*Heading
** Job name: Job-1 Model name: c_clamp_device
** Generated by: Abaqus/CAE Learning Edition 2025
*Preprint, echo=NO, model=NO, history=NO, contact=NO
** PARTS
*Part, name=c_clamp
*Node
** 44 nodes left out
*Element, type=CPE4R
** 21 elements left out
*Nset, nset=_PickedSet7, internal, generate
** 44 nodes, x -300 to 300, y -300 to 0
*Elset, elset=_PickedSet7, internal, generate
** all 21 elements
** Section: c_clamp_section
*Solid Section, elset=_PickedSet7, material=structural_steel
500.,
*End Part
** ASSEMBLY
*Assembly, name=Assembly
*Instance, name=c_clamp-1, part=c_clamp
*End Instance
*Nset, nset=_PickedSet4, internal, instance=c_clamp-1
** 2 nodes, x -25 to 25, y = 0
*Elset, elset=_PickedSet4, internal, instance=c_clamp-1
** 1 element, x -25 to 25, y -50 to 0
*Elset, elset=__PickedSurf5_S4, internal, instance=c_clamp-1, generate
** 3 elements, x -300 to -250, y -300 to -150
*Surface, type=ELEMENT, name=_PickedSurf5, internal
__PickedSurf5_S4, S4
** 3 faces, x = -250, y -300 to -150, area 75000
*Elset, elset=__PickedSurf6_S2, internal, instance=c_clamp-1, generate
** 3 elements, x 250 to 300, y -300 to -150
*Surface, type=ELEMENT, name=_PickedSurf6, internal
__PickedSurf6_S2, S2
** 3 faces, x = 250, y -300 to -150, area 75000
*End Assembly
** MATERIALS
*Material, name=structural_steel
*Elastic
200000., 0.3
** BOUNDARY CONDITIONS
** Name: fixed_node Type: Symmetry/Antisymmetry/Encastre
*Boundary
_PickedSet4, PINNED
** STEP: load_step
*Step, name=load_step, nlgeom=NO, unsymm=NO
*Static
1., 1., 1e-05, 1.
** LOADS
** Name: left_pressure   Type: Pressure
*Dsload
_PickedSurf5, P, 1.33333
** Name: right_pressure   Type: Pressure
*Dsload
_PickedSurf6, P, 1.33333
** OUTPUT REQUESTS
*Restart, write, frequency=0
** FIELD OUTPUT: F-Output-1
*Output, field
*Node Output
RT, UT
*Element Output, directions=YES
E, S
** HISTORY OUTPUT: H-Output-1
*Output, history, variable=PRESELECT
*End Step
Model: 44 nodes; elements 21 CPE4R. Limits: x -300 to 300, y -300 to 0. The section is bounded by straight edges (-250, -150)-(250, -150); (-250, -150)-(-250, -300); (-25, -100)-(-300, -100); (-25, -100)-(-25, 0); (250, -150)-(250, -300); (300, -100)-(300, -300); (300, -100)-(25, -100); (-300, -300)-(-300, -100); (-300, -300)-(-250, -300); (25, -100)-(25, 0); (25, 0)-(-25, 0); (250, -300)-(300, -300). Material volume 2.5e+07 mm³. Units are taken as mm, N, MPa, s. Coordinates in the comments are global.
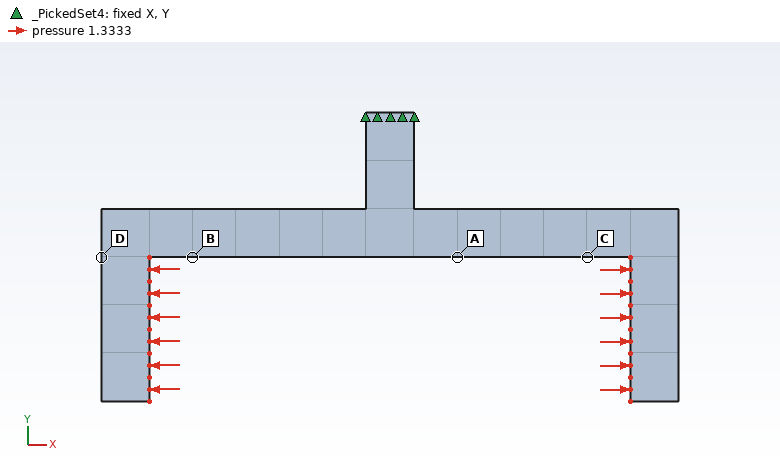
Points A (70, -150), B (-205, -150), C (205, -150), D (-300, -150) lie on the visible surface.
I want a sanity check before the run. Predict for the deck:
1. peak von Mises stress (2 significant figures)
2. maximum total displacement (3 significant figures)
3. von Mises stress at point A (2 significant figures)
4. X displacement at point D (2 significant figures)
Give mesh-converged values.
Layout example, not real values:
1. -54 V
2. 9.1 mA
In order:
1. 51 MPa
2. 0.595 mm
3. 46 MPa
4. -0.062 mm
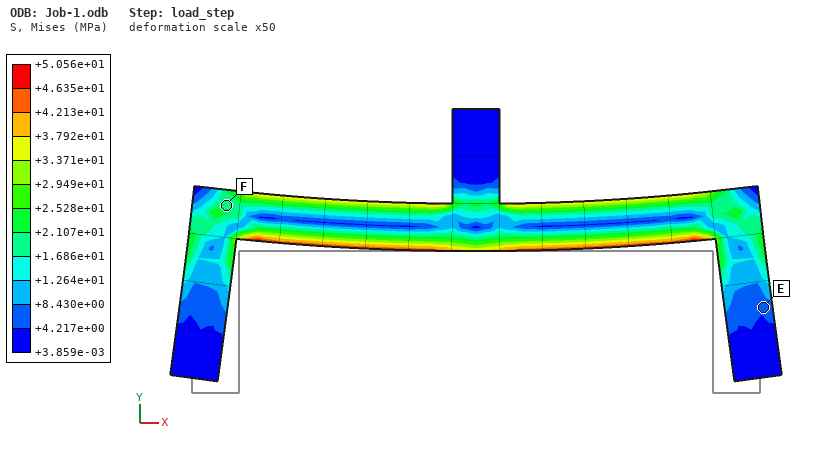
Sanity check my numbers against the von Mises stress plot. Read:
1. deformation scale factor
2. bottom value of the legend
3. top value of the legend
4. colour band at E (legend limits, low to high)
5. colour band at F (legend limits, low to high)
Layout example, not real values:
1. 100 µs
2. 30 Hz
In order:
1. 50
2. +3.859e-03 MPa
3. +5.056e+01 MPa
4. +4.217e+00 to +8.430e+00 MPa
5. +1.686e+01 to +2.107e+01 MPa
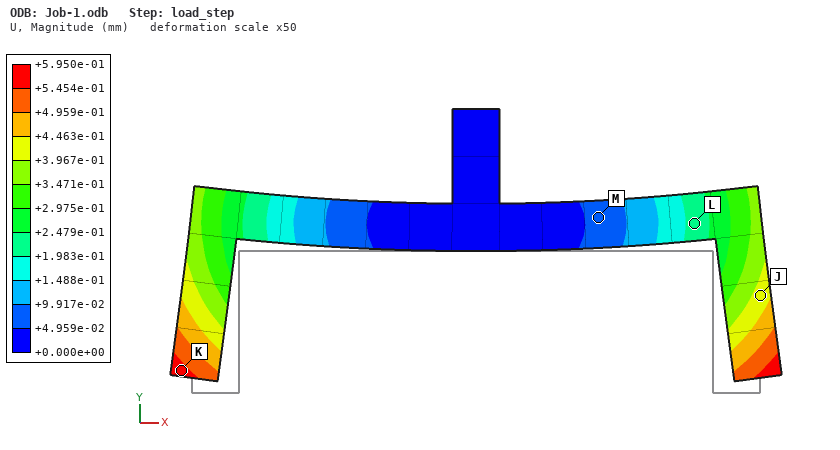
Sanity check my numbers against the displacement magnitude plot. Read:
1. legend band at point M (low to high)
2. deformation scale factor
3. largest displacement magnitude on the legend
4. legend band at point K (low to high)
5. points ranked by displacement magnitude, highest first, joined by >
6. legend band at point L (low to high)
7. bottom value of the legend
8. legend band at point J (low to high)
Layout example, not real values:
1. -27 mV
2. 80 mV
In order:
1. +4.959e-02 to +9.917e-02 mm
2. 50
3. +5.950e-01 mm
4. +5.454e-01 to +5.950e-01 mm
5. K > J > L > M
6. +1.983e-01 to +2.479e-01 mm
7. +0.000e+00 mm
8. +3.967e-01 to +4.463e-01 mm
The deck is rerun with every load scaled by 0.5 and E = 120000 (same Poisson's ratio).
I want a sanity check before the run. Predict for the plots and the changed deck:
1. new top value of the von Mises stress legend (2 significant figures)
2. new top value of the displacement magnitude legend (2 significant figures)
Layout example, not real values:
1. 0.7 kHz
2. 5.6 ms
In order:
1. 25 MPa
2. 0.50 mm
